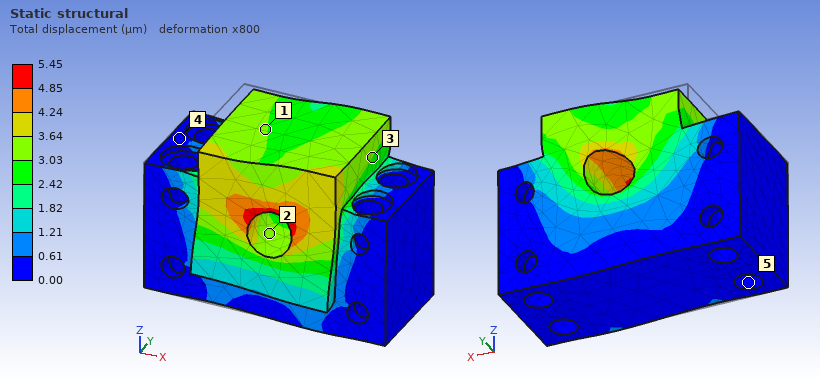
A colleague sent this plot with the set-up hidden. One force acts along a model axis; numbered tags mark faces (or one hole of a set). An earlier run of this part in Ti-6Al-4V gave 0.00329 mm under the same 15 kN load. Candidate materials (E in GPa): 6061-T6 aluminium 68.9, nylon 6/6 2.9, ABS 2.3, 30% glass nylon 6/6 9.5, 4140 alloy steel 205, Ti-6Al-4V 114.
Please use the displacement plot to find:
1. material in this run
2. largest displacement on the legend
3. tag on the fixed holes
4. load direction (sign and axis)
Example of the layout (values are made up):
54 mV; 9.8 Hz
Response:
6061-T6 aluminium; 5.45 µm; 5; +X
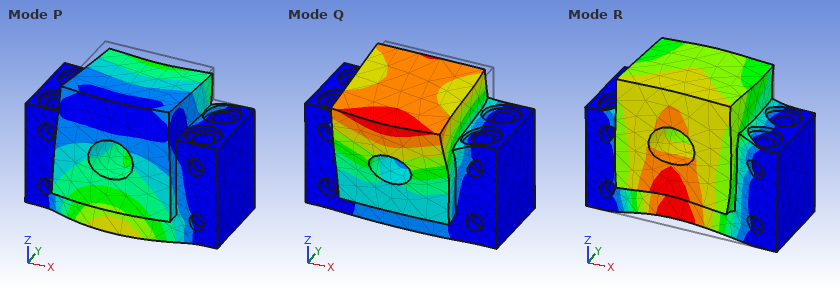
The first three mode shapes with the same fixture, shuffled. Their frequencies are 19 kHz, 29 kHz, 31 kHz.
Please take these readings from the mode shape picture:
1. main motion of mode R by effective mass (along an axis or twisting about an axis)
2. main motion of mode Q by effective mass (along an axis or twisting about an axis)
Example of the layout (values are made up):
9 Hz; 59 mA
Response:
along Z; along Y
